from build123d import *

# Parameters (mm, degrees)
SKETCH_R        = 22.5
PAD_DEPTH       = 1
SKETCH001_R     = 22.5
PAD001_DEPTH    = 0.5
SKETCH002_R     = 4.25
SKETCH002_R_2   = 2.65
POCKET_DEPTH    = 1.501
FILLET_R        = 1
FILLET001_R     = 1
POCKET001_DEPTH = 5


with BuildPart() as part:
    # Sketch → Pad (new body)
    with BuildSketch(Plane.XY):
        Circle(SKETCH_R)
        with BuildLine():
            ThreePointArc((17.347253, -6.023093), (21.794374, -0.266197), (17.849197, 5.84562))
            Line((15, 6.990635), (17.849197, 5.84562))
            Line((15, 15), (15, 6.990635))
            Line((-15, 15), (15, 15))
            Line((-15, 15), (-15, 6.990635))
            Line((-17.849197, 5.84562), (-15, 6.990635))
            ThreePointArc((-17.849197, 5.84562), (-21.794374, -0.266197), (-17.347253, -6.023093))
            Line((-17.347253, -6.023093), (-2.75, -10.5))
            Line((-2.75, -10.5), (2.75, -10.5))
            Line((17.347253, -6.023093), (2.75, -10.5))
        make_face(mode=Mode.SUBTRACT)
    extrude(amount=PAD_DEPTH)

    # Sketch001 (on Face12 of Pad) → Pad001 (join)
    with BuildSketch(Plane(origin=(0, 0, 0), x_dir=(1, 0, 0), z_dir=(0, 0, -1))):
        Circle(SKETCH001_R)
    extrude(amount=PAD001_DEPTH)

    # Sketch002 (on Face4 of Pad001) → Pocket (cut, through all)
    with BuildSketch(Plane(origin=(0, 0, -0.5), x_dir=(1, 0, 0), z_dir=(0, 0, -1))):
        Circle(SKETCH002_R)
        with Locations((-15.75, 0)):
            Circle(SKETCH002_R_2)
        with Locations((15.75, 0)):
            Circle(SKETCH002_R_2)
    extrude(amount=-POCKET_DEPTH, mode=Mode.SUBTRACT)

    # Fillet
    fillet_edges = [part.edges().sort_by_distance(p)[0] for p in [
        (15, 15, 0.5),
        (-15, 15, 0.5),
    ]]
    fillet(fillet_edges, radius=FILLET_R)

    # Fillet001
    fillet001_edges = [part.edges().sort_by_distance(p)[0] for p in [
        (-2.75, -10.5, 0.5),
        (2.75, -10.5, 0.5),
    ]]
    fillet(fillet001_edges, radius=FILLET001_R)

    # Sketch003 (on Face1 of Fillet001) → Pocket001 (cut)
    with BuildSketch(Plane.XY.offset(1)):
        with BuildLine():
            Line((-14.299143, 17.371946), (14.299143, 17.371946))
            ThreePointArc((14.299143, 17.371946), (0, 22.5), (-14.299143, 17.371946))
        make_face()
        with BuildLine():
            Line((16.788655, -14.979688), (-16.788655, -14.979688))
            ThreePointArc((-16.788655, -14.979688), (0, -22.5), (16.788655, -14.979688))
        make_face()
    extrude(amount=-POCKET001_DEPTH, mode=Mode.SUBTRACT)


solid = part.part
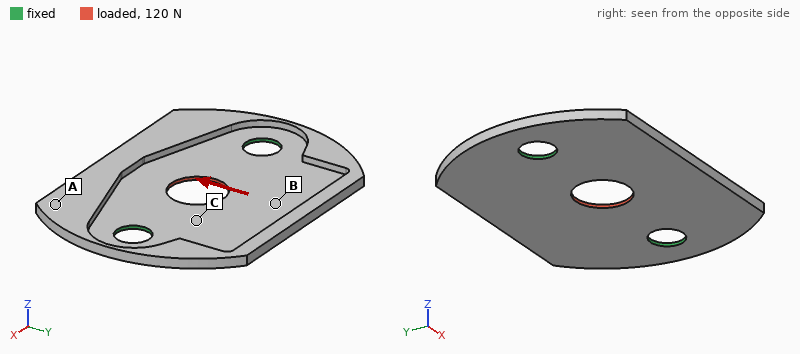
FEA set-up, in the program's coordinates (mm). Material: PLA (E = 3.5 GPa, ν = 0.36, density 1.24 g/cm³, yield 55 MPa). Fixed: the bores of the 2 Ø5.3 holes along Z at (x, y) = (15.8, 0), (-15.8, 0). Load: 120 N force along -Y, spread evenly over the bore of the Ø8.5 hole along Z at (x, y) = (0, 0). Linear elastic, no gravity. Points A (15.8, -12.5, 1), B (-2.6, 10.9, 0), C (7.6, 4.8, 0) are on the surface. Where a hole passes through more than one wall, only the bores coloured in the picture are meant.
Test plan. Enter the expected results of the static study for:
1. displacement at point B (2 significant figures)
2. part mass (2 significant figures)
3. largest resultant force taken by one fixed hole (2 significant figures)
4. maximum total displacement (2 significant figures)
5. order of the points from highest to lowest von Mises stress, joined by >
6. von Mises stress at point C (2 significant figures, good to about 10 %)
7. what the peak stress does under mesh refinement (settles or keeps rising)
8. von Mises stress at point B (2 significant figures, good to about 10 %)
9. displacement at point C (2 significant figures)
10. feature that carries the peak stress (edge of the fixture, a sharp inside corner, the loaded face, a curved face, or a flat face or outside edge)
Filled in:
0.062 mm
1.3 g
60 N
0.13 mm
C > B > A
9.0 MPa
keeps rising
6.0 MPa
0.035 mm
edge of the fixture
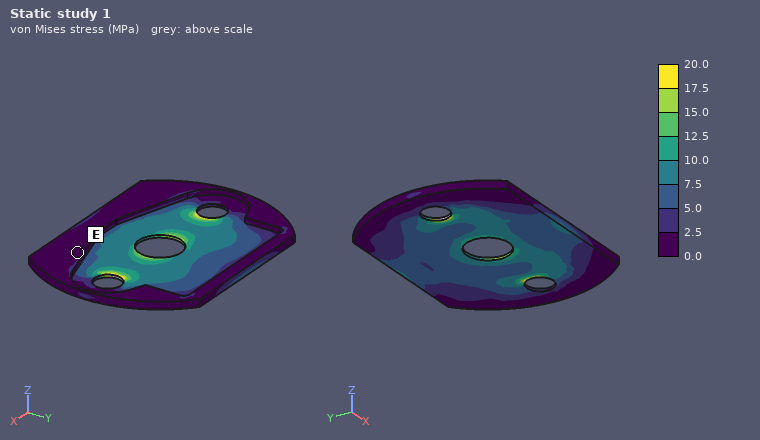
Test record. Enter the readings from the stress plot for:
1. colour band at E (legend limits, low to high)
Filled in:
0.0 to 2.5 MPa
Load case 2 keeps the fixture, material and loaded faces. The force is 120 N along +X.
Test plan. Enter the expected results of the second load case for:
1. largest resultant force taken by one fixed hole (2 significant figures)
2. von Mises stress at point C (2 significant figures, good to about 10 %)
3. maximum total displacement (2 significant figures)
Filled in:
60 N
6.8 MPa
40 µm
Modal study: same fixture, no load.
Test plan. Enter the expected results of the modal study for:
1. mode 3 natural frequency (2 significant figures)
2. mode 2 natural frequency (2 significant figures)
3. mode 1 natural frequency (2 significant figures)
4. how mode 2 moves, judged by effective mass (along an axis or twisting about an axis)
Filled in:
1100 Hz
700 Hz
600 Hz
along Z
